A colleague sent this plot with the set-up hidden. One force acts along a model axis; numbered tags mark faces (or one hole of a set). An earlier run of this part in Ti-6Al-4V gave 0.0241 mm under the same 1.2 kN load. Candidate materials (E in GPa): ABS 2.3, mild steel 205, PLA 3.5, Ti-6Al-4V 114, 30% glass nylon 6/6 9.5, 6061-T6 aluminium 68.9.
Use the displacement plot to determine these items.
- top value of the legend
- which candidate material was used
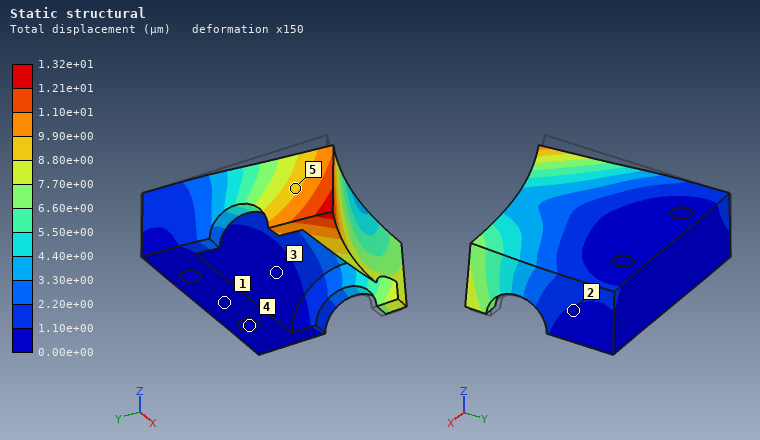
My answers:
1.32e+01 µm
mild steel
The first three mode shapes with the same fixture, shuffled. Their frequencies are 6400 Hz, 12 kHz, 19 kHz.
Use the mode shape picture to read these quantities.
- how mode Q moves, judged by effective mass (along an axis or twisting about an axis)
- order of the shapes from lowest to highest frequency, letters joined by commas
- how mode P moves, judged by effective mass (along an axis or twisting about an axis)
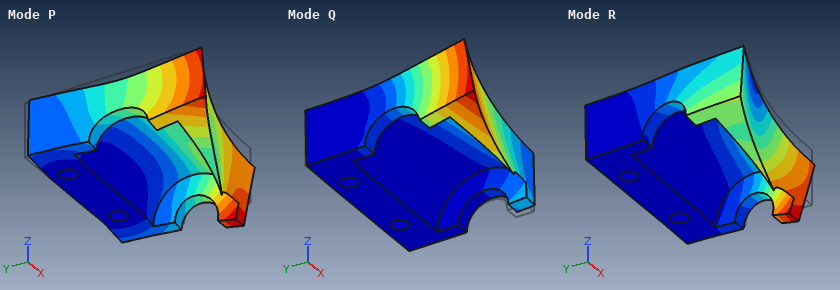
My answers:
along Z
Q, R, P
along X
